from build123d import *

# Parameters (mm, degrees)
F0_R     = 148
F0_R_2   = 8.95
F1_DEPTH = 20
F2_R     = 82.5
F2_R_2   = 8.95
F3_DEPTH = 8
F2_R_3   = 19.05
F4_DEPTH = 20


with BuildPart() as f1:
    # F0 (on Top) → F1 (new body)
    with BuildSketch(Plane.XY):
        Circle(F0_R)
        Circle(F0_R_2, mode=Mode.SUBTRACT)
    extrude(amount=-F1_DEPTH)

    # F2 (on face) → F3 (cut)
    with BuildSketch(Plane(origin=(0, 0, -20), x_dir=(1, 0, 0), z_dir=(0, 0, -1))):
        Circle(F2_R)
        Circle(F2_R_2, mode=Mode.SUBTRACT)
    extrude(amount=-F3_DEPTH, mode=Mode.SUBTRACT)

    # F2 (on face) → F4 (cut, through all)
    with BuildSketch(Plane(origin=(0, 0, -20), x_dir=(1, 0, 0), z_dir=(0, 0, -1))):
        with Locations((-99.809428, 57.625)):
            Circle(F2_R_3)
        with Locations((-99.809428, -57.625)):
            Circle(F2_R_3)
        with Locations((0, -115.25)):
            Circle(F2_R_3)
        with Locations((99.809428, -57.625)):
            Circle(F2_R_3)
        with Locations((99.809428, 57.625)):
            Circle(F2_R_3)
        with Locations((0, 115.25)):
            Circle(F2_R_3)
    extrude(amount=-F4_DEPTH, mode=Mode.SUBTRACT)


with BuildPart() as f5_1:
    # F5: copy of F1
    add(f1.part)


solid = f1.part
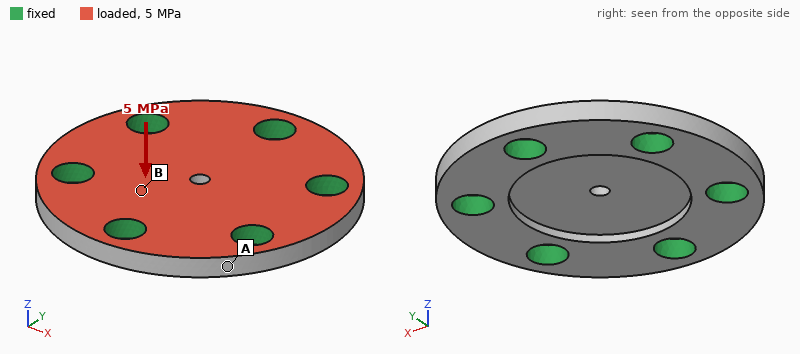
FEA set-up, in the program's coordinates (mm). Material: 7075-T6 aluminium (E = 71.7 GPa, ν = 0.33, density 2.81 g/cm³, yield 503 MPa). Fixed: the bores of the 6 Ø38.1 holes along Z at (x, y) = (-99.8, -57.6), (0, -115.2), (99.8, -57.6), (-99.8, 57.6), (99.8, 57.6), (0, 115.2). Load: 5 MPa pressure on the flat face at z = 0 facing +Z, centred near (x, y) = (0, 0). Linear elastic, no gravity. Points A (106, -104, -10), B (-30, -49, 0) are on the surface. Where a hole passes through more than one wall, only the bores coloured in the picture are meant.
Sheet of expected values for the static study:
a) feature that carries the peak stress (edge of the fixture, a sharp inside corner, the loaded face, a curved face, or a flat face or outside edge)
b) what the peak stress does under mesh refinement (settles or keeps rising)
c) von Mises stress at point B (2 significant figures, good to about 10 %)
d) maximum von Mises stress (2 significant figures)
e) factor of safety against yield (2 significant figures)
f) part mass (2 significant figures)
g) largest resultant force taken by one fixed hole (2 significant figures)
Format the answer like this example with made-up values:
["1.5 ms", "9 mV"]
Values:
["the loaded face", "settles", "74 MPa", "280 MPa", "1.8", "3.0 kg", "52 kN"]
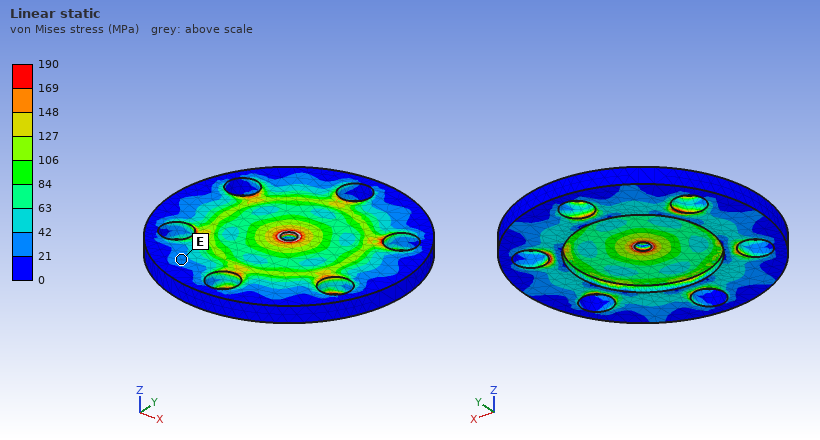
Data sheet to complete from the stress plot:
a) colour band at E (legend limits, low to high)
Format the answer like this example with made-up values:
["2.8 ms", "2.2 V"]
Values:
["21 to 42 MPa"]
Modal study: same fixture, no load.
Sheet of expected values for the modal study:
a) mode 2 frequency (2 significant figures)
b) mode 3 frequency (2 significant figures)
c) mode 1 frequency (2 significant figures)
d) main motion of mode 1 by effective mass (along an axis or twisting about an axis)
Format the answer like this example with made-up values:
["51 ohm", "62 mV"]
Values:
["6300 Hz", "6300 Hz", "3300 Hz", "along Z"]
